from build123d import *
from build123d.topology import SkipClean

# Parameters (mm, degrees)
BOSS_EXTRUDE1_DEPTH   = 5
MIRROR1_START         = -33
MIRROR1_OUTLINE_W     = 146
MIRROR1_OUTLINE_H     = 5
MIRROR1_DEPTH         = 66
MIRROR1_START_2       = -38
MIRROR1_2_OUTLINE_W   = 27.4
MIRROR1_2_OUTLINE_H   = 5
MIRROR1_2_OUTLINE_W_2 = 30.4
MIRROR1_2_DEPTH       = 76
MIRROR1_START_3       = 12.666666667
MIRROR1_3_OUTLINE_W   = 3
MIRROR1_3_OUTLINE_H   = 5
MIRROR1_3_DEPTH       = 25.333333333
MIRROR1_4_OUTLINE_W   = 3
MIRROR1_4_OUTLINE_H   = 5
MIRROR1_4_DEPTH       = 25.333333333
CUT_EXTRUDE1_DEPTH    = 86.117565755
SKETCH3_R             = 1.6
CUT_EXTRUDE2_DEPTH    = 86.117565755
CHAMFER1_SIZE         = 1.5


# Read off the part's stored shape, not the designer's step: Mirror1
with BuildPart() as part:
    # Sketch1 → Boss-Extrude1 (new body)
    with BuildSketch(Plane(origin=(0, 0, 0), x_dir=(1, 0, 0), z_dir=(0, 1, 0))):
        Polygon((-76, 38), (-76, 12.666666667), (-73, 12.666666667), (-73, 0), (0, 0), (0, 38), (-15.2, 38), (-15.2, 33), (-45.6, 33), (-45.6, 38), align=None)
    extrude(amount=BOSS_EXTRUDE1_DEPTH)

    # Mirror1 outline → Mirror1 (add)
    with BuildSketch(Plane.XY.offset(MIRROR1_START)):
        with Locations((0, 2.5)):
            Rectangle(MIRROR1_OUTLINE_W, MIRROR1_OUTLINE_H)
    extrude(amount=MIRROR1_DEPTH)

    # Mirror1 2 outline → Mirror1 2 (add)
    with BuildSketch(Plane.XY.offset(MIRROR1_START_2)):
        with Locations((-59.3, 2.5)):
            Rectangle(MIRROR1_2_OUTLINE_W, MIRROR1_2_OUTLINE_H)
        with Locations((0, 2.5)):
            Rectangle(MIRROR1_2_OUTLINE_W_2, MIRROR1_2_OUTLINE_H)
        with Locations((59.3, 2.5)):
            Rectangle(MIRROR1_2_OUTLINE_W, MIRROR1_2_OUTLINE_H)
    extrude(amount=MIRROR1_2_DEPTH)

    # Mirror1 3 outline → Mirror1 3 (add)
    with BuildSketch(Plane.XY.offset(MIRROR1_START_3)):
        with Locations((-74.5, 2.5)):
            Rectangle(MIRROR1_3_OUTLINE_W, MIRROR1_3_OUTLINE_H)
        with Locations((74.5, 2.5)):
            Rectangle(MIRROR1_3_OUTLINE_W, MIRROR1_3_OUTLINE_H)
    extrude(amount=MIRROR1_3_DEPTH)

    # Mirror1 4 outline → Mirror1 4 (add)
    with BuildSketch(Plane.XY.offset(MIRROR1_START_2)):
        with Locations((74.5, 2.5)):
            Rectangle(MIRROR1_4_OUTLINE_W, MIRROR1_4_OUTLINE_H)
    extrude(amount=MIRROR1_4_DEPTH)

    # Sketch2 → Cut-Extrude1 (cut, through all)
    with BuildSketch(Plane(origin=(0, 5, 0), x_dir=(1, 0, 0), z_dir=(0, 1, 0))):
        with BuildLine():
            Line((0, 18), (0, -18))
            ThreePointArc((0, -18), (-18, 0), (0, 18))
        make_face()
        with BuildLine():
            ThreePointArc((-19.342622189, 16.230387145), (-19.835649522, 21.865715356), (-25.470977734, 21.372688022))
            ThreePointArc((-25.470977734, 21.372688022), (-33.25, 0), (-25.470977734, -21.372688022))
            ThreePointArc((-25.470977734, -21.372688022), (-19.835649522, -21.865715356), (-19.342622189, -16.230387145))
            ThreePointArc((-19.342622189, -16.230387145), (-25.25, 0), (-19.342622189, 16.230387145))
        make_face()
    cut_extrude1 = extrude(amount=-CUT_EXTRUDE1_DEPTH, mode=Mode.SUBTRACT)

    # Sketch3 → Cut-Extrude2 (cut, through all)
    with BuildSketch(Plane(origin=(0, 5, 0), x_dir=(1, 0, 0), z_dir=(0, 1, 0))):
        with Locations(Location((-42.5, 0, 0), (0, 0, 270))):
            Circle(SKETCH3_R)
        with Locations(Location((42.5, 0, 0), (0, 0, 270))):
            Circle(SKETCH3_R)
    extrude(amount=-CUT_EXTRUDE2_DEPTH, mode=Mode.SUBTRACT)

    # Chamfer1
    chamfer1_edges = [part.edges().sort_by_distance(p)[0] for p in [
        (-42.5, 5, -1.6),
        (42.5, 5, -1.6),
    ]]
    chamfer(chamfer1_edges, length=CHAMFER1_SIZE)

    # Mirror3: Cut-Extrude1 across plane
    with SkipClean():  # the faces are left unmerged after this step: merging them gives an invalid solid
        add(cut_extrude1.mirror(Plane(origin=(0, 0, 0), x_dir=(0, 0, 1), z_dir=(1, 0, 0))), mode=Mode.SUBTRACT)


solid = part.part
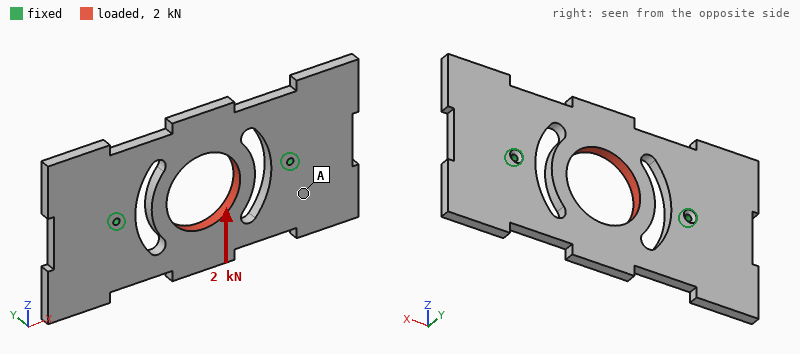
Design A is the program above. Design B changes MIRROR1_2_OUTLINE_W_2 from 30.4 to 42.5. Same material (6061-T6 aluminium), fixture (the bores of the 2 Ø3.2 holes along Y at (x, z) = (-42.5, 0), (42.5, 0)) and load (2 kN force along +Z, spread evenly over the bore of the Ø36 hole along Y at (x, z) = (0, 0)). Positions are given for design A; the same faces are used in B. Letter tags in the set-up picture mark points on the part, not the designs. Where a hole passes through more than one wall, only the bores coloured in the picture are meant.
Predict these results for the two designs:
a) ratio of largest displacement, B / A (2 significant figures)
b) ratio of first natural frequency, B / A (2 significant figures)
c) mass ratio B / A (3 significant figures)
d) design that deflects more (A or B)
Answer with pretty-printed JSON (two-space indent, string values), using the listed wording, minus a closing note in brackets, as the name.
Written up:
{
  "ratio of largest displacement, B / A": "0.91",
  "ratio of first natural frequency, B / A": "0.98",
  "mass ratio B / A": "1.01",
  "design that deflects more": "A"
}
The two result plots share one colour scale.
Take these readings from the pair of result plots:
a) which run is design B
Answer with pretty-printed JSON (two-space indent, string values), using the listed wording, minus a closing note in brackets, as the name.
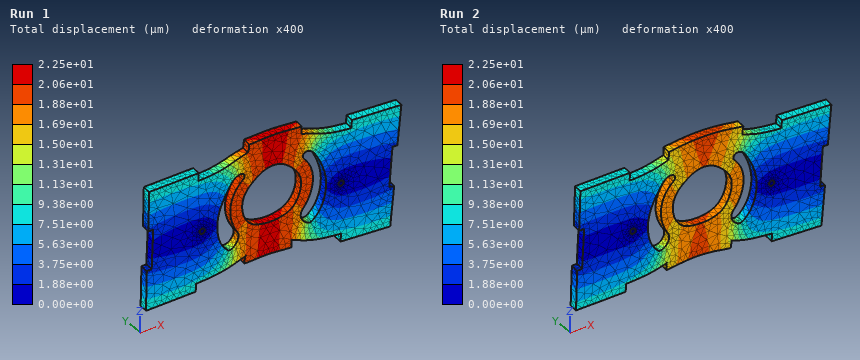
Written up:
{
  "which run is design B": "Run 2"
}
